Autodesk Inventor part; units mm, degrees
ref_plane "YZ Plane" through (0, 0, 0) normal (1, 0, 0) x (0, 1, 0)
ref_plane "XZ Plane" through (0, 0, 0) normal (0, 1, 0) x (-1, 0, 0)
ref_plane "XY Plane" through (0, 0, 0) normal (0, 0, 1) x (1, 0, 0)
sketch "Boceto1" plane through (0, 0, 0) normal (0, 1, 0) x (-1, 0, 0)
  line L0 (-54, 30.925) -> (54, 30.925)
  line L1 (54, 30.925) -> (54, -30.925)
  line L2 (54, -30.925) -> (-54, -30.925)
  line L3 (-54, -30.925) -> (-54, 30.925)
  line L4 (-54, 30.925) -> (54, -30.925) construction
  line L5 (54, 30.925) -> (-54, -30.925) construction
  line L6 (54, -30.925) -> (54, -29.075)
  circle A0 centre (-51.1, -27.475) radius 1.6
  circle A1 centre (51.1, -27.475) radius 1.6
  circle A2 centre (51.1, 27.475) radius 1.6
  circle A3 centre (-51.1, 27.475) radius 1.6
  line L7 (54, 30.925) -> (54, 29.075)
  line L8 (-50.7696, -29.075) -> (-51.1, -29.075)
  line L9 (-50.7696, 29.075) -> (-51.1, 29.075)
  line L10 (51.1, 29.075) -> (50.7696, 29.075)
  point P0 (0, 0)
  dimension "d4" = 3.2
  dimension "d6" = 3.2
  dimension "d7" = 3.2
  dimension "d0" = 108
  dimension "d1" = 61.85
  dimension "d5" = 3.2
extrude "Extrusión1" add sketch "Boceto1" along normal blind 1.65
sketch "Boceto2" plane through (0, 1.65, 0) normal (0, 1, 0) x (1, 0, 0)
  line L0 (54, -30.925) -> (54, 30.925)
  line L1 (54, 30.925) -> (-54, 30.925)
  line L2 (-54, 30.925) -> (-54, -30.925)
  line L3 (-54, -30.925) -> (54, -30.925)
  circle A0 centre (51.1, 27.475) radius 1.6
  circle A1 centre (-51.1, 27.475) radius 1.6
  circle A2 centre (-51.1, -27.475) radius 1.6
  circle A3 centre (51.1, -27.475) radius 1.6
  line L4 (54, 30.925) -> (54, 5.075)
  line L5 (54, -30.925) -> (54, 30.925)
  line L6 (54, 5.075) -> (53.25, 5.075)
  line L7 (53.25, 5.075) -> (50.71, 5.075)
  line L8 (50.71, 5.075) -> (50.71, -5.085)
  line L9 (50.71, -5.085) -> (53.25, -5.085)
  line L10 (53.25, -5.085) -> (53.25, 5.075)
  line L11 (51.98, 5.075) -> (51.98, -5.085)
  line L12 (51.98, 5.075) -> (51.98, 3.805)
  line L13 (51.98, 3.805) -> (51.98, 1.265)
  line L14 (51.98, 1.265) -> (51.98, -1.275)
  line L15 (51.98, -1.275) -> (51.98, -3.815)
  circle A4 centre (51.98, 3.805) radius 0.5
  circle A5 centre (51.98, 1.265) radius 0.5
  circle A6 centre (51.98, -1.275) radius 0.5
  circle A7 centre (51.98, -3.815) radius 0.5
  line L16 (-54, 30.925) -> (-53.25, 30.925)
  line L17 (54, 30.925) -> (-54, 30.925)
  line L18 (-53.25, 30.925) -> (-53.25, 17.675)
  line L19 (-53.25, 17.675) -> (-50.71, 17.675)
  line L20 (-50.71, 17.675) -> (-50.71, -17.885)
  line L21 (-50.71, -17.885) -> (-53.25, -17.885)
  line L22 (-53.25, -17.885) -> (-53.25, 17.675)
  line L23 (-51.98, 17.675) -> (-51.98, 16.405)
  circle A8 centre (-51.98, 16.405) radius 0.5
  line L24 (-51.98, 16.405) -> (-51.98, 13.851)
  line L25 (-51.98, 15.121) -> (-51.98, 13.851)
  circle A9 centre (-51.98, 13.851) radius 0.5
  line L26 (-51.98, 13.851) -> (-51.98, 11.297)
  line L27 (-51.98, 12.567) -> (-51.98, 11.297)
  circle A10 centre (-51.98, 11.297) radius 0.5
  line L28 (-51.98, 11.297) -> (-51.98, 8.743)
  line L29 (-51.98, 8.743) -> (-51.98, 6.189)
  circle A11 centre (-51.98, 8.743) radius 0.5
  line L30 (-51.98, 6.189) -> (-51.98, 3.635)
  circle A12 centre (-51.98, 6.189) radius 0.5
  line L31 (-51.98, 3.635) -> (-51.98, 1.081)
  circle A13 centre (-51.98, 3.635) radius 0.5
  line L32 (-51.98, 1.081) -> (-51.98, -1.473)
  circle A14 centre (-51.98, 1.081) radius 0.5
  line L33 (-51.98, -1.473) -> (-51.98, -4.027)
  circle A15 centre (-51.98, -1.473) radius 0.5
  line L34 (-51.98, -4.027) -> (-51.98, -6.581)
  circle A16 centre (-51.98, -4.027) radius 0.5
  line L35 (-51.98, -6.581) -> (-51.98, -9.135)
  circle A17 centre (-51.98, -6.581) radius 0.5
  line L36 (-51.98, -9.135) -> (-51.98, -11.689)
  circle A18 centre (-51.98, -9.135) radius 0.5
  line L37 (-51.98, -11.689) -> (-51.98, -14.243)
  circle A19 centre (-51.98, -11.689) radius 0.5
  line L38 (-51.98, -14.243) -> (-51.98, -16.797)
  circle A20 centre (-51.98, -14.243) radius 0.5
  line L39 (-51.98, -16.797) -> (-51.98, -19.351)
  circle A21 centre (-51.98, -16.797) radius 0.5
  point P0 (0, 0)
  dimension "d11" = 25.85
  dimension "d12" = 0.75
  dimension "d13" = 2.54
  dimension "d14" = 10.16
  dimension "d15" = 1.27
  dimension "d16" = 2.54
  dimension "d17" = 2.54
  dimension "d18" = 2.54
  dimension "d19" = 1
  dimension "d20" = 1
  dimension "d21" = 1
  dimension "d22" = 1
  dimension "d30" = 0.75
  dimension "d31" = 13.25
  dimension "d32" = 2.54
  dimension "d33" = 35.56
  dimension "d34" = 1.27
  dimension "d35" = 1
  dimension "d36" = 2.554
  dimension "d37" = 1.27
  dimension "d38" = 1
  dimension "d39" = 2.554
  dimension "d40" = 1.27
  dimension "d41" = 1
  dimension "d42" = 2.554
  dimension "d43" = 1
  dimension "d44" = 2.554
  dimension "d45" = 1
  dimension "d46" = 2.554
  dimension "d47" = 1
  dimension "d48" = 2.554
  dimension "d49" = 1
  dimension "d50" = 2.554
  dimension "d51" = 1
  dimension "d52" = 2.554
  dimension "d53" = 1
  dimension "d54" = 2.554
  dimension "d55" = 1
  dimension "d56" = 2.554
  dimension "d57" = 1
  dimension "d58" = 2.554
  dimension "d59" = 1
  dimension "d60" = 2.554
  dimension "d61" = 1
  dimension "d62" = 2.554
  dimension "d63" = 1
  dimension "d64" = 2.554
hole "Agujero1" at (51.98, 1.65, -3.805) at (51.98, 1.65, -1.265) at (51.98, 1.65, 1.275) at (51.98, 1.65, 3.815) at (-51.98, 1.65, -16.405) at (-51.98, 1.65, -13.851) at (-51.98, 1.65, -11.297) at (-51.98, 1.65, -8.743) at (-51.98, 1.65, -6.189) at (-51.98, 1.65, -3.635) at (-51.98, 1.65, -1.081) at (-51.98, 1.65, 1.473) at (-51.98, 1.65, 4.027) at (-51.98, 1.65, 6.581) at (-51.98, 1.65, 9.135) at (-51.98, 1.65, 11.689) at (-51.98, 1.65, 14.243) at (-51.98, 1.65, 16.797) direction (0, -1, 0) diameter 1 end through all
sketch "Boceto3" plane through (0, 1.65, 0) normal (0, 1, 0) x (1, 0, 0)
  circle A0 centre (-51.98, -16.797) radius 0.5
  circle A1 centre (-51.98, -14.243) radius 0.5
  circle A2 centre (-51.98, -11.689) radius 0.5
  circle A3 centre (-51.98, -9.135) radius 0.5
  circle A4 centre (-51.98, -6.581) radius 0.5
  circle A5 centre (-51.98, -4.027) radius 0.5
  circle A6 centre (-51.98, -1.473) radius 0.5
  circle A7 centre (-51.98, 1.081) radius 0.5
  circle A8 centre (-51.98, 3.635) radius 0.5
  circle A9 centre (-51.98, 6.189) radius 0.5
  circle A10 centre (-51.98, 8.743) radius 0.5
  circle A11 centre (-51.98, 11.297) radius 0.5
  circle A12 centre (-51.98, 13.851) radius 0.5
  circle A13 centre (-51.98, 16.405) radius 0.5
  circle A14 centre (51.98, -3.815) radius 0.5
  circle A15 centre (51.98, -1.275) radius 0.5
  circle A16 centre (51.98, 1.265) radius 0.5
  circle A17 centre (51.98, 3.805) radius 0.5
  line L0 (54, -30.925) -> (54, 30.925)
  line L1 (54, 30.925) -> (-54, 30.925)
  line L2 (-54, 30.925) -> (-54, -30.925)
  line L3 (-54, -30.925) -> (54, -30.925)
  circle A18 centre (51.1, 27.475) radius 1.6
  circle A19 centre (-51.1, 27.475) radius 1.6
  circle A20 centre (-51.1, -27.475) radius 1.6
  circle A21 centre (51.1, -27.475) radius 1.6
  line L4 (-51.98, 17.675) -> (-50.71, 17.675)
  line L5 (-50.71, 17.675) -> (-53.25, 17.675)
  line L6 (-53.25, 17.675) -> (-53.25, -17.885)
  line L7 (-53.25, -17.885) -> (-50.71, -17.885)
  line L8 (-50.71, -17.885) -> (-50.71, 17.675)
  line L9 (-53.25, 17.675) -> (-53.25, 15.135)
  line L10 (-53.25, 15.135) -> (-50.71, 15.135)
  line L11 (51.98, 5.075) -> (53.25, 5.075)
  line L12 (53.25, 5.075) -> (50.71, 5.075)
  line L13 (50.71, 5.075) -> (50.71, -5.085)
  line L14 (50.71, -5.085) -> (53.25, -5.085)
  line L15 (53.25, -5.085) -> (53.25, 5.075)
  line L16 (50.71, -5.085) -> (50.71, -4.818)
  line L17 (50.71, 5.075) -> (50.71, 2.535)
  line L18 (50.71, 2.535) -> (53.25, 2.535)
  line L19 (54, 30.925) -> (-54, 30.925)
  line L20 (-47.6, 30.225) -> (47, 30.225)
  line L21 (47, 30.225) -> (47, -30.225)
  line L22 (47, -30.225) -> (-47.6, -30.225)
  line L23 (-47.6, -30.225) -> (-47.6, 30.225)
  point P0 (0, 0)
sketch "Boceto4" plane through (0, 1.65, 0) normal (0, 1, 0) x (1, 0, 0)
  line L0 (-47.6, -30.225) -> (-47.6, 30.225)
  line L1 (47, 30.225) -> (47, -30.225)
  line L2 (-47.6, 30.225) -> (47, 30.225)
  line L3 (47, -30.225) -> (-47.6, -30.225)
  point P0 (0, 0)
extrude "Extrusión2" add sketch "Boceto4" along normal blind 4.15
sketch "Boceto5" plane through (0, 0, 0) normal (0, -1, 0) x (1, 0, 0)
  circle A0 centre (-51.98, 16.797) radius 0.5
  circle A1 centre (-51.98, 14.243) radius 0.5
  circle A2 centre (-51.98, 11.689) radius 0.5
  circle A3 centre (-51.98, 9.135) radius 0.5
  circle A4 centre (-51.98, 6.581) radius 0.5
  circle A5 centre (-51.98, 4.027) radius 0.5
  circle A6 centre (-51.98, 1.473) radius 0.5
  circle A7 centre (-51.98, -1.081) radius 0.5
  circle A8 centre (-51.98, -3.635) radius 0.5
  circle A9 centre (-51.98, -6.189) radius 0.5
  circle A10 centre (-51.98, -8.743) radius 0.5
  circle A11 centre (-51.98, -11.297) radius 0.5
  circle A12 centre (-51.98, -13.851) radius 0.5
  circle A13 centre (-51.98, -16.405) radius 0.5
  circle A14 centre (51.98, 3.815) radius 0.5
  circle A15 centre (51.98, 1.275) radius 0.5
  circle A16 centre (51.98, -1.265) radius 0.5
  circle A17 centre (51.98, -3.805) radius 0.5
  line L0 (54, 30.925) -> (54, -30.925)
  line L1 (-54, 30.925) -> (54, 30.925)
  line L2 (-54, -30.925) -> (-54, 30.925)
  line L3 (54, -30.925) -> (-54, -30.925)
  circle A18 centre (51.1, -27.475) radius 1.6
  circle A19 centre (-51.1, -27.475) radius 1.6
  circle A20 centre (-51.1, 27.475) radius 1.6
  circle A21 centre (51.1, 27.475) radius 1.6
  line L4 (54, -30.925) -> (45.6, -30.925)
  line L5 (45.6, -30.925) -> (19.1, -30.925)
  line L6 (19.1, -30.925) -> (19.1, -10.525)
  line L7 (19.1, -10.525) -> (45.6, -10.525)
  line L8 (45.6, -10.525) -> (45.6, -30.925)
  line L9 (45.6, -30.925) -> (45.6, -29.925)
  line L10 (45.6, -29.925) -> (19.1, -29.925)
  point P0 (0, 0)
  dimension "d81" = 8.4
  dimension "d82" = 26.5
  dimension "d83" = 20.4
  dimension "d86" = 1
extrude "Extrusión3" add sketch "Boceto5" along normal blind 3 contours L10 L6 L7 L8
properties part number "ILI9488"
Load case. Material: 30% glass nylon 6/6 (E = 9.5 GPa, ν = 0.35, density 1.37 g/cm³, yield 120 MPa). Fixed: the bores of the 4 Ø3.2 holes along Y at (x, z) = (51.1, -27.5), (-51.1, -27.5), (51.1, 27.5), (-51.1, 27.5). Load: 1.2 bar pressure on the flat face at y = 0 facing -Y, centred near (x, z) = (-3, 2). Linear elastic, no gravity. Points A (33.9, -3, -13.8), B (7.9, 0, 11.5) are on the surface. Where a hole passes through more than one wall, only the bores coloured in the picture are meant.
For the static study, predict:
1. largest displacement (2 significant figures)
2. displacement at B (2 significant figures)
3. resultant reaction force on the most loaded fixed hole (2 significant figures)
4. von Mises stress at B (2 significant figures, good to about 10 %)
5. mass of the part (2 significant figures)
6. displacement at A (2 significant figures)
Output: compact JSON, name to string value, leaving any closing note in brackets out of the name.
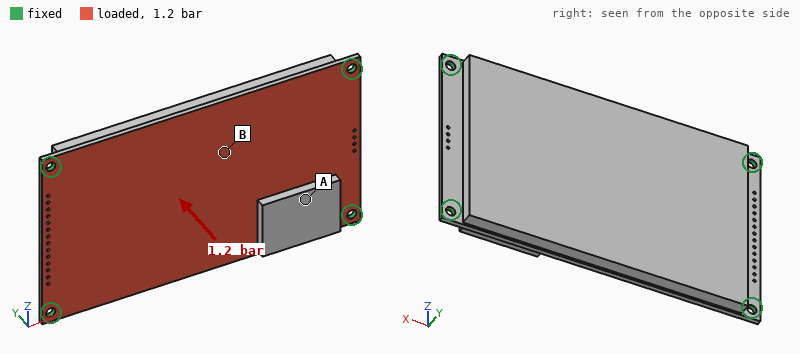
{"largest displacement": "0.66 mm", "displacement at B": "0.59 mm", "resultant reaction force on the most loaded fixed hole": "540 N", "von Mises stress at B": "12 MPa", "mass of the part": "50 g", "displacement at A": "0.30 mm"}
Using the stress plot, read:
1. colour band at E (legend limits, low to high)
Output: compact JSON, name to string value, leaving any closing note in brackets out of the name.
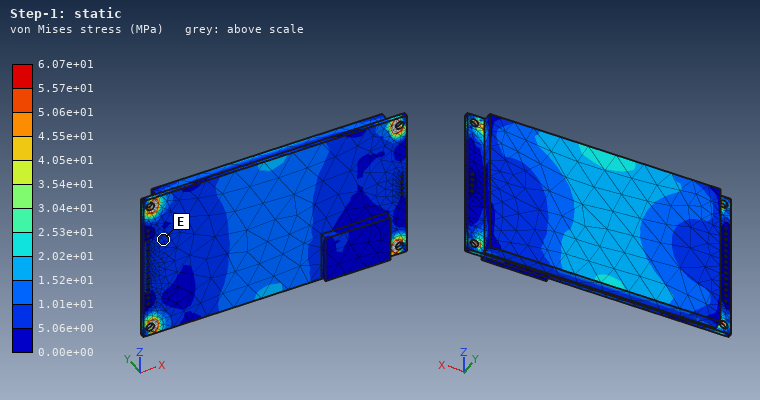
{"colour band at E": "5.06e+00 to 1.01e+01 MPa"}
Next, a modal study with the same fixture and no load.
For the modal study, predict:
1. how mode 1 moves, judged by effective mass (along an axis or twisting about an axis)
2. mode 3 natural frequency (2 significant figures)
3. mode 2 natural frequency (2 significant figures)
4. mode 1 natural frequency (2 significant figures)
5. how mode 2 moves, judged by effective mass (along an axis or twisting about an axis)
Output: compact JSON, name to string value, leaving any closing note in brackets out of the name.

{"how mode 1 moves, judged by effective mass": "along Y", "mode 3 natural frequency": "2300 Hz", "mode 2 natural frequency": "1700 Hz", "mode 1 natural frequency": "860 Hz", "how mode 2 moves, judged by effective mass": "twisting about X"}
